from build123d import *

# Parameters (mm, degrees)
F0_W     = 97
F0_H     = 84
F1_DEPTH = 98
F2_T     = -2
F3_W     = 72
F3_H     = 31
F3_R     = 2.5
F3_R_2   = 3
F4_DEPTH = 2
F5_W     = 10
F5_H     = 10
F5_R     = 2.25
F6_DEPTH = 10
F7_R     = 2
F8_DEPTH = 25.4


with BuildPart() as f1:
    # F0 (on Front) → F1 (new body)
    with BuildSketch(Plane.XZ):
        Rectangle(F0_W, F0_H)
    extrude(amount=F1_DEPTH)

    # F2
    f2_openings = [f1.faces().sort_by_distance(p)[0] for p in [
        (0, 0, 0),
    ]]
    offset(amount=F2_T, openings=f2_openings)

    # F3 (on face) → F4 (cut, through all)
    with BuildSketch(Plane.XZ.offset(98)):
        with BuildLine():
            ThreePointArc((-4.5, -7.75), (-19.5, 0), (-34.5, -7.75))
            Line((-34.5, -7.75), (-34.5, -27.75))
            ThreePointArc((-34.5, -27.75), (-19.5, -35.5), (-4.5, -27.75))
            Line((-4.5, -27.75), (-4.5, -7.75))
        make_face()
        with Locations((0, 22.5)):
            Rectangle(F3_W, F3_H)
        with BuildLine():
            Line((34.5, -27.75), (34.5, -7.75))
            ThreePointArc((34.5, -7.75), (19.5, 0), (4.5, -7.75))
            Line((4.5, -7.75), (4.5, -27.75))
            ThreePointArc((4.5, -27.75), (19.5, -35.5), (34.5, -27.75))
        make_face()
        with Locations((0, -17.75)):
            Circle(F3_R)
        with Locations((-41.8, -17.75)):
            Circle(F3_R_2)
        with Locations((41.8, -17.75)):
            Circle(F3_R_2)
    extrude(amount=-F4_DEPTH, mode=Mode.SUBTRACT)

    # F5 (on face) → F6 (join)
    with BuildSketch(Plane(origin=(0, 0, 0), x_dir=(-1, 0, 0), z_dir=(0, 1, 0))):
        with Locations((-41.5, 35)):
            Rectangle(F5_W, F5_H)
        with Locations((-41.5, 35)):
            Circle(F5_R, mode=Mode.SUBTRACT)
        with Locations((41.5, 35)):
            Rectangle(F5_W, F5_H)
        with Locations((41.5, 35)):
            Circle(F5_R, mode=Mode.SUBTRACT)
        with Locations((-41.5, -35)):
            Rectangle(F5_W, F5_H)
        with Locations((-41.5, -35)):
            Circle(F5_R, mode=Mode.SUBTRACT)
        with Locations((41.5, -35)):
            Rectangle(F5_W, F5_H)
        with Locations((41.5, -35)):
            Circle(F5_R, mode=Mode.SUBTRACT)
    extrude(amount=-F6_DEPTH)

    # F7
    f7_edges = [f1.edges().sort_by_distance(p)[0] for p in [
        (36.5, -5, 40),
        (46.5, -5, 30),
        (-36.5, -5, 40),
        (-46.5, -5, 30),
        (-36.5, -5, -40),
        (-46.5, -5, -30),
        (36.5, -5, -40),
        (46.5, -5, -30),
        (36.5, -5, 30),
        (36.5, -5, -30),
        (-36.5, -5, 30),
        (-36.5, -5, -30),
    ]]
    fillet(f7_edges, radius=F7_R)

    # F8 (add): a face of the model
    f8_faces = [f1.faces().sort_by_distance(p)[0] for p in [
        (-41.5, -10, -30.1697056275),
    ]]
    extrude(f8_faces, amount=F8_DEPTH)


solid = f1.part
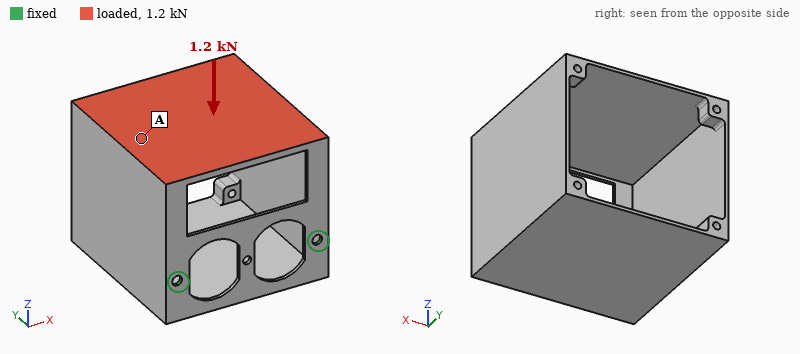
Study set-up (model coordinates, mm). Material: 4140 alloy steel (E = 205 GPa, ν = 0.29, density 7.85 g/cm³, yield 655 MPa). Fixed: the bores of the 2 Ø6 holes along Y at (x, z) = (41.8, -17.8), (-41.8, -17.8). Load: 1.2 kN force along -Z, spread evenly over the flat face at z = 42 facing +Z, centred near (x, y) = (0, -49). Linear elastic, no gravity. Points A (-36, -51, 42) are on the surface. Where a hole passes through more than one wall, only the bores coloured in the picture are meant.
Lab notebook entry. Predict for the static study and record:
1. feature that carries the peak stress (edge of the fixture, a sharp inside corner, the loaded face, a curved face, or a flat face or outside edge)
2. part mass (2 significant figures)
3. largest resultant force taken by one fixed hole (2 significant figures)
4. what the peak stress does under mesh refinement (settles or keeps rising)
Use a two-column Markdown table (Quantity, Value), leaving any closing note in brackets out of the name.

| Quantity | Value |
|---|---|
| feature that carries the peak stress | edge of the fixture |
| part mass | 640 g |
| largest resultant force taken by one fixed hole | 600 N |
| what the peak stress does under mesh refinement | keeps rising |
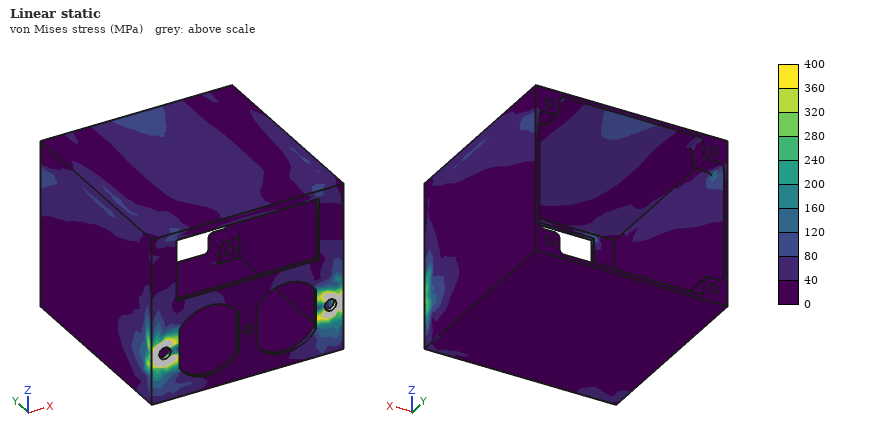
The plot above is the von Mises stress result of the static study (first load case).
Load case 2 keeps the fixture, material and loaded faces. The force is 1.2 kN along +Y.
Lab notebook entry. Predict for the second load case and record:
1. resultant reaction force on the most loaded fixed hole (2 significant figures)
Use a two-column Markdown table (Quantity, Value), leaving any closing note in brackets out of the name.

| Quantity | Value |
|---|---|
| resultant reaction force on the most loaded fixed hole | 600 N |
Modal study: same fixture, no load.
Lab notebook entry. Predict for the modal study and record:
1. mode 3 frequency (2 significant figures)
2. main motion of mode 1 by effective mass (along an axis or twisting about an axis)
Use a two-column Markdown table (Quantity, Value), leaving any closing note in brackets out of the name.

| Quantity | Value |
|---|---|
| mode 3 frequency | 740 Hz |
| main motion of mode 1 by effective mass | along Z |
